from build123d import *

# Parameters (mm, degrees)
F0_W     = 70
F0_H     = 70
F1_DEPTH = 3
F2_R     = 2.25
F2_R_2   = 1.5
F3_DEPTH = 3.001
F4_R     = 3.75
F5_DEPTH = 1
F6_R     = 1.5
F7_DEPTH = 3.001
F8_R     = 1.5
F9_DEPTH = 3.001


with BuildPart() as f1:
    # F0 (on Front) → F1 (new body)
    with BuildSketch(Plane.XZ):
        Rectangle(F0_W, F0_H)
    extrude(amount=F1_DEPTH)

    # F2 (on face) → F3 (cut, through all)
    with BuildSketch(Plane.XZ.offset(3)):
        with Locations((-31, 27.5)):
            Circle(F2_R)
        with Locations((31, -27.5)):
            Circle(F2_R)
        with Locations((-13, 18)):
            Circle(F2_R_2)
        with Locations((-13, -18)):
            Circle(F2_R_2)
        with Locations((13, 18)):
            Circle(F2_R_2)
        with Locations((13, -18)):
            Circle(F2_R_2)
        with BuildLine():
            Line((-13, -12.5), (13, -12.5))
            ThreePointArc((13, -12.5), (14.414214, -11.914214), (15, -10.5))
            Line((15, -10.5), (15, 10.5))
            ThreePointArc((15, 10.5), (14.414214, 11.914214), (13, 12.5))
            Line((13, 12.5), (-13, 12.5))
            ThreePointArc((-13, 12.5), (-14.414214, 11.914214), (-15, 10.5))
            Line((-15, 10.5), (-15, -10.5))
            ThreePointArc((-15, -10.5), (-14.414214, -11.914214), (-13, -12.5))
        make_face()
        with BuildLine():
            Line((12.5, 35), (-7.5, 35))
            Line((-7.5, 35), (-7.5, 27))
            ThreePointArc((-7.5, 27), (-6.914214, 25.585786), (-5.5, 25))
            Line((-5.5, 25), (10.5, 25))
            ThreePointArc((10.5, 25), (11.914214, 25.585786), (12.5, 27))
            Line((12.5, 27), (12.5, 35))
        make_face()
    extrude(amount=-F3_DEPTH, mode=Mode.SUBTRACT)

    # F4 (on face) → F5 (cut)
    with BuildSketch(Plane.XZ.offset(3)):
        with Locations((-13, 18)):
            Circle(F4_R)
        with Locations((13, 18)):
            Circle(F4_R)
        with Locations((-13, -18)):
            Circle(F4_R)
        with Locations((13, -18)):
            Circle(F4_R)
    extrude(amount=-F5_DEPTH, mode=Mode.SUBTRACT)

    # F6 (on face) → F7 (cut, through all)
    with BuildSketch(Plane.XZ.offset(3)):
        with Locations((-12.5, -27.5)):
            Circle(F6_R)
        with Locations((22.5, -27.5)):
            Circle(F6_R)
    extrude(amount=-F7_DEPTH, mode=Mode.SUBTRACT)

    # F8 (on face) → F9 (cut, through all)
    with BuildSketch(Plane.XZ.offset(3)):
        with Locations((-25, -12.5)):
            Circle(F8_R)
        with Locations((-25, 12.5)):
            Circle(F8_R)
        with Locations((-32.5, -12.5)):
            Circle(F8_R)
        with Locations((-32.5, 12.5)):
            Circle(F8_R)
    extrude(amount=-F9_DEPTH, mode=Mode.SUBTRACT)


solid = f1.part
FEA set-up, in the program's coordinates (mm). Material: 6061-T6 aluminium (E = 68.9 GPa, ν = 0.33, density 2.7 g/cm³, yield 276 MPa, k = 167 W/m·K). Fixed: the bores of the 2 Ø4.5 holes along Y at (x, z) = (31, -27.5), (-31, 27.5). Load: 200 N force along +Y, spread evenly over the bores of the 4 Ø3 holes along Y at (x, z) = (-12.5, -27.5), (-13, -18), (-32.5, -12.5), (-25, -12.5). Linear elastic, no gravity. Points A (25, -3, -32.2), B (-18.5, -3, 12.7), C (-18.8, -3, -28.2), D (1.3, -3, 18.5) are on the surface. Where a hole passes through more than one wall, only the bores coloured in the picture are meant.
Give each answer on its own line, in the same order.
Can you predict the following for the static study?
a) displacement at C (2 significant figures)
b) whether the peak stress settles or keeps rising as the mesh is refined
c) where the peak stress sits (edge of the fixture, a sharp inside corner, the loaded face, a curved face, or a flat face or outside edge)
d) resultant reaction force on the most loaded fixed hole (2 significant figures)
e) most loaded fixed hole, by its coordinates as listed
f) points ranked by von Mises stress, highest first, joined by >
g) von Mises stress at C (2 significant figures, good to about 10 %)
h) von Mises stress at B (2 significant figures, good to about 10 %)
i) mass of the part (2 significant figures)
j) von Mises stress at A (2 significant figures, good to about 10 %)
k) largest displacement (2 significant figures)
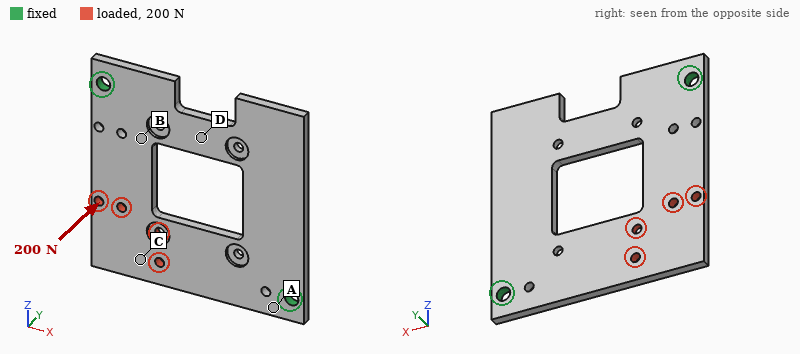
0.63 mm
keeps rising
edge of the fixture
120 N
(-31, 27.5)
A > B > C > D
36 MPa
69 MPa
31 g
97 MPa
0.94 mm
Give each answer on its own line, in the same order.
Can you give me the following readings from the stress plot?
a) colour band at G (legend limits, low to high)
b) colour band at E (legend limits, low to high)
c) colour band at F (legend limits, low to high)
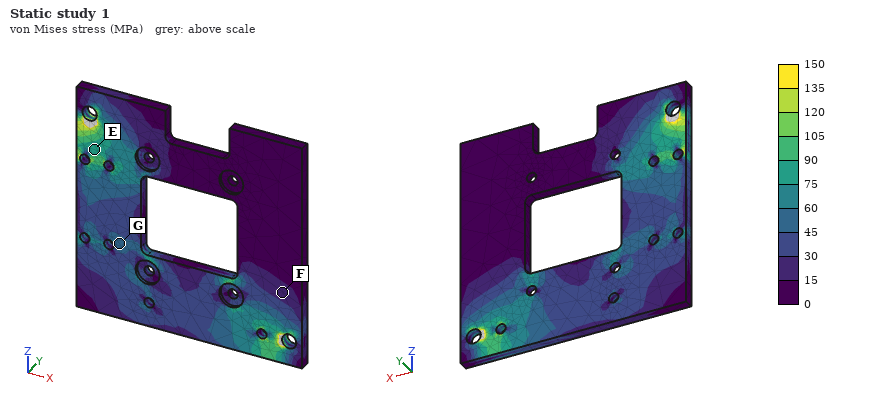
45 to 60 MPa
75 to 90 MPa
15 to 30 MPa
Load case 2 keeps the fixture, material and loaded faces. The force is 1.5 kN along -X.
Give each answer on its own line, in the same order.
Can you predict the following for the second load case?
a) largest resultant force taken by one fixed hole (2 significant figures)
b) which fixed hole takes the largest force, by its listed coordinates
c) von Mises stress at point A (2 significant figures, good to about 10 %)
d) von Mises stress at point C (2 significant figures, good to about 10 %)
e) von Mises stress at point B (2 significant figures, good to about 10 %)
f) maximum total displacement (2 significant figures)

1.2 kN
(31, -27.5)
24 MPa
7.2 MPa
6.8 MPa
24 µm
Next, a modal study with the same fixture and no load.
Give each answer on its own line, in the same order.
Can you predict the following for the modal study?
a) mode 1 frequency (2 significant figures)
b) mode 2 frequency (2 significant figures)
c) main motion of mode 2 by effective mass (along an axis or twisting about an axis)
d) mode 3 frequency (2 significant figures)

900 Hz
1100 Hz
along Y
3200 Hz
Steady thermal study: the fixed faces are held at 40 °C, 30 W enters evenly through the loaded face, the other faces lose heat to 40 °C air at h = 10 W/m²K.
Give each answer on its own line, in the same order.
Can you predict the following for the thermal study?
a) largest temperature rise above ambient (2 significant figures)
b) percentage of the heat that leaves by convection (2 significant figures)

68 K
8.3 %
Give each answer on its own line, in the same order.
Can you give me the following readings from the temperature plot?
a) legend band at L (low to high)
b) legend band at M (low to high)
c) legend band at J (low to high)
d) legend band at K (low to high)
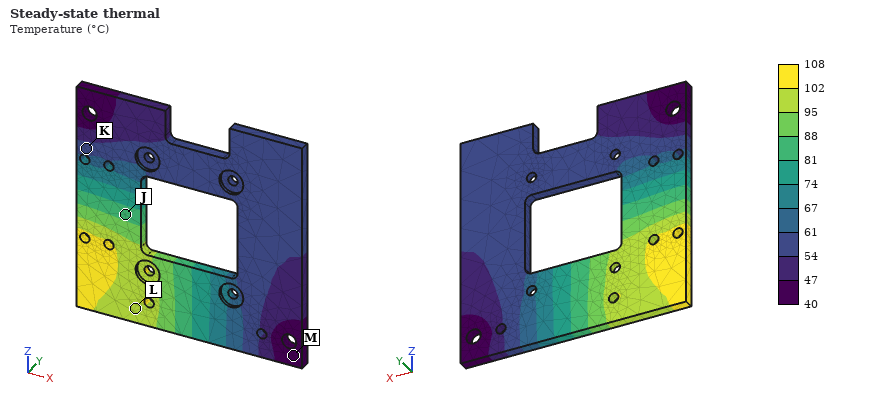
95 to 102 °C
40 to 47 °C
81 to 88 °C
54 to 61 °C
